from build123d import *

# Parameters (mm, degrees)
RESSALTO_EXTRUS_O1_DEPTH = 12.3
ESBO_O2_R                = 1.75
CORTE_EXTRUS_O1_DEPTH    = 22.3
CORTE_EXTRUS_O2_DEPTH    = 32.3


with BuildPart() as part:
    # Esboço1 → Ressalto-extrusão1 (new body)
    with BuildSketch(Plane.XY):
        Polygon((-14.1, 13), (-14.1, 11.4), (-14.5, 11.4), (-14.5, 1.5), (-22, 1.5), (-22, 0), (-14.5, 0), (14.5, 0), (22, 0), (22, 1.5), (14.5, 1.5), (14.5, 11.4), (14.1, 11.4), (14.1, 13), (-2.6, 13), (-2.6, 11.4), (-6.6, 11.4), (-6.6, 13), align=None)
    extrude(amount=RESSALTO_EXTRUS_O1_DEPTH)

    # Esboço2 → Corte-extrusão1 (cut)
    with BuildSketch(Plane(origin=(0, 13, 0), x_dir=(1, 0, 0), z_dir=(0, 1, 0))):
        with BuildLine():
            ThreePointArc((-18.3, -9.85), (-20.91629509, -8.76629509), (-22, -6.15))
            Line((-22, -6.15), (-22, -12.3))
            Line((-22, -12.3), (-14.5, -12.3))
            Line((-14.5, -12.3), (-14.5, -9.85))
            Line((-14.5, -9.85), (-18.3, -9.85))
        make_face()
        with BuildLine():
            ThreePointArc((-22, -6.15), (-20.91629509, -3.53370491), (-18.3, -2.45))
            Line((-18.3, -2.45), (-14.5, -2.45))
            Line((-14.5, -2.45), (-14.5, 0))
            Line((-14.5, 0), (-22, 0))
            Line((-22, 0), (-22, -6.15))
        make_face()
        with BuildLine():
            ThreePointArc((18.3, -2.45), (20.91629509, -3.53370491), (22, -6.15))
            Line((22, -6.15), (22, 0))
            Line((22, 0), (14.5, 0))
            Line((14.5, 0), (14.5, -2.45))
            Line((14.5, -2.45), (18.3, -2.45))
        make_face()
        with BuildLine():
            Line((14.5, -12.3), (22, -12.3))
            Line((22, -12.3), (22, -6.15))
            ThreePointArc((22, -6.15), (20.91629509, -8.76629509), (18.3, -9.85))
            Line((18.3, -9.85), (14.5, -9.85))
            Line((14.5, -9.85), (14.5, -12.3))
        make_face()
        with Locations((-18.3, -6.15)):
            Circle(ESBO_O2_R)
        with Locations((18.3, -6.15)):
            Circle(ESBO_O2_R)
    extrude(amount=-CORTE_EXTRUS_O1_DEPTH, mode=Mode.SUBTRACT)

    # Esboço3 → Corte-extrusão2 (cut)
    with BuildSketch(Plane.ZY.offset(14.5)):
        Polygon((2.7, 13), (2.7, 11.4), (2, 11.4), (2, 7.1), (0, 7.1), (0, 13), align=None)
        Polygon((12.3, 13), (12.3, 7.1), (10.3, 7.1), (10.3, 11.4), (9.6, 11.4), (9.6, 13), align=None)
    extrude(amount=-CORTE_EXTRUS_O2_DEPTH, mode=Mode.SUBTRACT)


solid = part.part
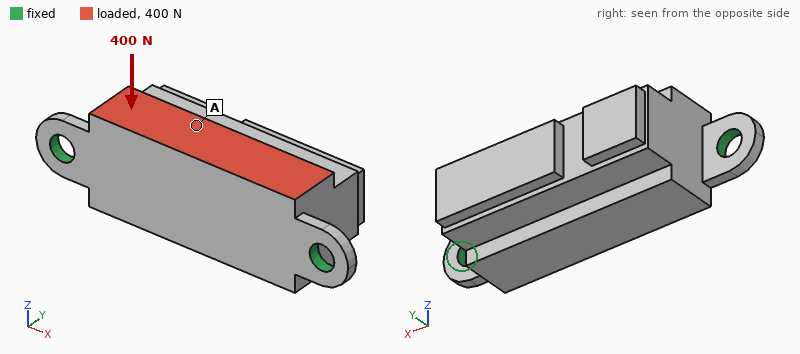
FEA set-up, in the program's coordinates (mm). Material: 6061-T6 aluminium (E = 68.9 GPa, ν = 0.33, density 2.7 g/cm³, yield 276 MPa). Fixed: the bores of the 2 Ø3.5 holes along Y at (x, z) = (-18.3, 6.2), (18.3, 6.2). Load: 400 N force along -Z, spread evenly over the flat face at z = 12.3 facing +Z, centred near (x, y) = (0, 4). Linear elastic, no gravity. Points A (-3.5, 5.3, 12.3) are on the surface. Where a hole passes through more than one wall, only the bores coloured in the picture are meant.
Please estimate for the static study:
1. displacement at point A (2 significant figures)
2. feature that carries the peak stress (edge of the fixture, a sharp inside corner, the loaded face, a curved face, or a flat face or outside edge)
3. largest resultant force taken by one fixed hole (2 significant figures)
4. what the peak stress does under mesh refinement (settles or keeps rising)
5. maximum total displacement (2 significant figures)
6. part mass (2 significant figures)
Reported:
38 µm
edge of the fixture
200 N
keeps rising
63 µm
11 g
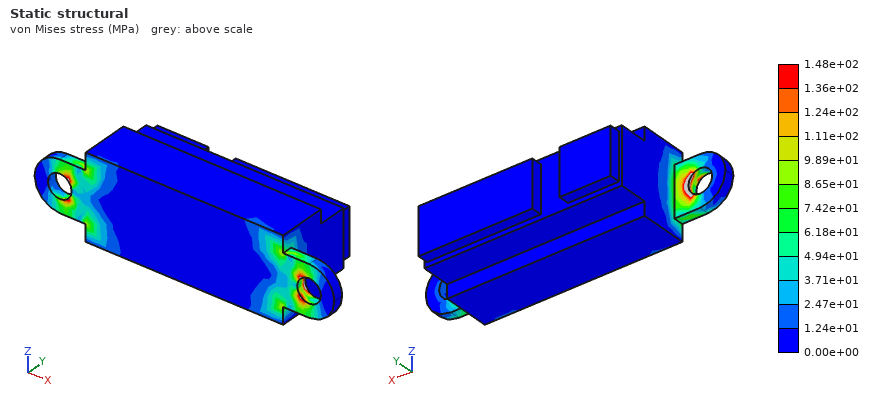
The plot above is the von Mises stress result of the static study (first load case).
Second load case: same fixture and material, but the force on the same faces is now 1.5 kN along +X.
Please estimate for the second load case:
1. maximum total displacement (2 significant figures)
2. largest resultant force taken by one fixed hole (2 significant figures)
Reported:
12 µm
810 N
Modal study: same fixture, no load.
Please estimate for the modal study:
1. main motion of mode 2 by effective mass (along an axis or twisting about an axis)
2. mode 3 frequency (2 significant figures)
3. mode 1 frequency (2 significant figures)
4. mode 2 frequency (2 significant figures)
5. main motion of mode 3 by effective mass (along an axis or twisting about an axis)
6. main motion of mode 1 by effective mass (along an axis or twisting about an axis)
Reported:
along Y
17 kHz
3500 Hz
11 kHz
along X
along Z
